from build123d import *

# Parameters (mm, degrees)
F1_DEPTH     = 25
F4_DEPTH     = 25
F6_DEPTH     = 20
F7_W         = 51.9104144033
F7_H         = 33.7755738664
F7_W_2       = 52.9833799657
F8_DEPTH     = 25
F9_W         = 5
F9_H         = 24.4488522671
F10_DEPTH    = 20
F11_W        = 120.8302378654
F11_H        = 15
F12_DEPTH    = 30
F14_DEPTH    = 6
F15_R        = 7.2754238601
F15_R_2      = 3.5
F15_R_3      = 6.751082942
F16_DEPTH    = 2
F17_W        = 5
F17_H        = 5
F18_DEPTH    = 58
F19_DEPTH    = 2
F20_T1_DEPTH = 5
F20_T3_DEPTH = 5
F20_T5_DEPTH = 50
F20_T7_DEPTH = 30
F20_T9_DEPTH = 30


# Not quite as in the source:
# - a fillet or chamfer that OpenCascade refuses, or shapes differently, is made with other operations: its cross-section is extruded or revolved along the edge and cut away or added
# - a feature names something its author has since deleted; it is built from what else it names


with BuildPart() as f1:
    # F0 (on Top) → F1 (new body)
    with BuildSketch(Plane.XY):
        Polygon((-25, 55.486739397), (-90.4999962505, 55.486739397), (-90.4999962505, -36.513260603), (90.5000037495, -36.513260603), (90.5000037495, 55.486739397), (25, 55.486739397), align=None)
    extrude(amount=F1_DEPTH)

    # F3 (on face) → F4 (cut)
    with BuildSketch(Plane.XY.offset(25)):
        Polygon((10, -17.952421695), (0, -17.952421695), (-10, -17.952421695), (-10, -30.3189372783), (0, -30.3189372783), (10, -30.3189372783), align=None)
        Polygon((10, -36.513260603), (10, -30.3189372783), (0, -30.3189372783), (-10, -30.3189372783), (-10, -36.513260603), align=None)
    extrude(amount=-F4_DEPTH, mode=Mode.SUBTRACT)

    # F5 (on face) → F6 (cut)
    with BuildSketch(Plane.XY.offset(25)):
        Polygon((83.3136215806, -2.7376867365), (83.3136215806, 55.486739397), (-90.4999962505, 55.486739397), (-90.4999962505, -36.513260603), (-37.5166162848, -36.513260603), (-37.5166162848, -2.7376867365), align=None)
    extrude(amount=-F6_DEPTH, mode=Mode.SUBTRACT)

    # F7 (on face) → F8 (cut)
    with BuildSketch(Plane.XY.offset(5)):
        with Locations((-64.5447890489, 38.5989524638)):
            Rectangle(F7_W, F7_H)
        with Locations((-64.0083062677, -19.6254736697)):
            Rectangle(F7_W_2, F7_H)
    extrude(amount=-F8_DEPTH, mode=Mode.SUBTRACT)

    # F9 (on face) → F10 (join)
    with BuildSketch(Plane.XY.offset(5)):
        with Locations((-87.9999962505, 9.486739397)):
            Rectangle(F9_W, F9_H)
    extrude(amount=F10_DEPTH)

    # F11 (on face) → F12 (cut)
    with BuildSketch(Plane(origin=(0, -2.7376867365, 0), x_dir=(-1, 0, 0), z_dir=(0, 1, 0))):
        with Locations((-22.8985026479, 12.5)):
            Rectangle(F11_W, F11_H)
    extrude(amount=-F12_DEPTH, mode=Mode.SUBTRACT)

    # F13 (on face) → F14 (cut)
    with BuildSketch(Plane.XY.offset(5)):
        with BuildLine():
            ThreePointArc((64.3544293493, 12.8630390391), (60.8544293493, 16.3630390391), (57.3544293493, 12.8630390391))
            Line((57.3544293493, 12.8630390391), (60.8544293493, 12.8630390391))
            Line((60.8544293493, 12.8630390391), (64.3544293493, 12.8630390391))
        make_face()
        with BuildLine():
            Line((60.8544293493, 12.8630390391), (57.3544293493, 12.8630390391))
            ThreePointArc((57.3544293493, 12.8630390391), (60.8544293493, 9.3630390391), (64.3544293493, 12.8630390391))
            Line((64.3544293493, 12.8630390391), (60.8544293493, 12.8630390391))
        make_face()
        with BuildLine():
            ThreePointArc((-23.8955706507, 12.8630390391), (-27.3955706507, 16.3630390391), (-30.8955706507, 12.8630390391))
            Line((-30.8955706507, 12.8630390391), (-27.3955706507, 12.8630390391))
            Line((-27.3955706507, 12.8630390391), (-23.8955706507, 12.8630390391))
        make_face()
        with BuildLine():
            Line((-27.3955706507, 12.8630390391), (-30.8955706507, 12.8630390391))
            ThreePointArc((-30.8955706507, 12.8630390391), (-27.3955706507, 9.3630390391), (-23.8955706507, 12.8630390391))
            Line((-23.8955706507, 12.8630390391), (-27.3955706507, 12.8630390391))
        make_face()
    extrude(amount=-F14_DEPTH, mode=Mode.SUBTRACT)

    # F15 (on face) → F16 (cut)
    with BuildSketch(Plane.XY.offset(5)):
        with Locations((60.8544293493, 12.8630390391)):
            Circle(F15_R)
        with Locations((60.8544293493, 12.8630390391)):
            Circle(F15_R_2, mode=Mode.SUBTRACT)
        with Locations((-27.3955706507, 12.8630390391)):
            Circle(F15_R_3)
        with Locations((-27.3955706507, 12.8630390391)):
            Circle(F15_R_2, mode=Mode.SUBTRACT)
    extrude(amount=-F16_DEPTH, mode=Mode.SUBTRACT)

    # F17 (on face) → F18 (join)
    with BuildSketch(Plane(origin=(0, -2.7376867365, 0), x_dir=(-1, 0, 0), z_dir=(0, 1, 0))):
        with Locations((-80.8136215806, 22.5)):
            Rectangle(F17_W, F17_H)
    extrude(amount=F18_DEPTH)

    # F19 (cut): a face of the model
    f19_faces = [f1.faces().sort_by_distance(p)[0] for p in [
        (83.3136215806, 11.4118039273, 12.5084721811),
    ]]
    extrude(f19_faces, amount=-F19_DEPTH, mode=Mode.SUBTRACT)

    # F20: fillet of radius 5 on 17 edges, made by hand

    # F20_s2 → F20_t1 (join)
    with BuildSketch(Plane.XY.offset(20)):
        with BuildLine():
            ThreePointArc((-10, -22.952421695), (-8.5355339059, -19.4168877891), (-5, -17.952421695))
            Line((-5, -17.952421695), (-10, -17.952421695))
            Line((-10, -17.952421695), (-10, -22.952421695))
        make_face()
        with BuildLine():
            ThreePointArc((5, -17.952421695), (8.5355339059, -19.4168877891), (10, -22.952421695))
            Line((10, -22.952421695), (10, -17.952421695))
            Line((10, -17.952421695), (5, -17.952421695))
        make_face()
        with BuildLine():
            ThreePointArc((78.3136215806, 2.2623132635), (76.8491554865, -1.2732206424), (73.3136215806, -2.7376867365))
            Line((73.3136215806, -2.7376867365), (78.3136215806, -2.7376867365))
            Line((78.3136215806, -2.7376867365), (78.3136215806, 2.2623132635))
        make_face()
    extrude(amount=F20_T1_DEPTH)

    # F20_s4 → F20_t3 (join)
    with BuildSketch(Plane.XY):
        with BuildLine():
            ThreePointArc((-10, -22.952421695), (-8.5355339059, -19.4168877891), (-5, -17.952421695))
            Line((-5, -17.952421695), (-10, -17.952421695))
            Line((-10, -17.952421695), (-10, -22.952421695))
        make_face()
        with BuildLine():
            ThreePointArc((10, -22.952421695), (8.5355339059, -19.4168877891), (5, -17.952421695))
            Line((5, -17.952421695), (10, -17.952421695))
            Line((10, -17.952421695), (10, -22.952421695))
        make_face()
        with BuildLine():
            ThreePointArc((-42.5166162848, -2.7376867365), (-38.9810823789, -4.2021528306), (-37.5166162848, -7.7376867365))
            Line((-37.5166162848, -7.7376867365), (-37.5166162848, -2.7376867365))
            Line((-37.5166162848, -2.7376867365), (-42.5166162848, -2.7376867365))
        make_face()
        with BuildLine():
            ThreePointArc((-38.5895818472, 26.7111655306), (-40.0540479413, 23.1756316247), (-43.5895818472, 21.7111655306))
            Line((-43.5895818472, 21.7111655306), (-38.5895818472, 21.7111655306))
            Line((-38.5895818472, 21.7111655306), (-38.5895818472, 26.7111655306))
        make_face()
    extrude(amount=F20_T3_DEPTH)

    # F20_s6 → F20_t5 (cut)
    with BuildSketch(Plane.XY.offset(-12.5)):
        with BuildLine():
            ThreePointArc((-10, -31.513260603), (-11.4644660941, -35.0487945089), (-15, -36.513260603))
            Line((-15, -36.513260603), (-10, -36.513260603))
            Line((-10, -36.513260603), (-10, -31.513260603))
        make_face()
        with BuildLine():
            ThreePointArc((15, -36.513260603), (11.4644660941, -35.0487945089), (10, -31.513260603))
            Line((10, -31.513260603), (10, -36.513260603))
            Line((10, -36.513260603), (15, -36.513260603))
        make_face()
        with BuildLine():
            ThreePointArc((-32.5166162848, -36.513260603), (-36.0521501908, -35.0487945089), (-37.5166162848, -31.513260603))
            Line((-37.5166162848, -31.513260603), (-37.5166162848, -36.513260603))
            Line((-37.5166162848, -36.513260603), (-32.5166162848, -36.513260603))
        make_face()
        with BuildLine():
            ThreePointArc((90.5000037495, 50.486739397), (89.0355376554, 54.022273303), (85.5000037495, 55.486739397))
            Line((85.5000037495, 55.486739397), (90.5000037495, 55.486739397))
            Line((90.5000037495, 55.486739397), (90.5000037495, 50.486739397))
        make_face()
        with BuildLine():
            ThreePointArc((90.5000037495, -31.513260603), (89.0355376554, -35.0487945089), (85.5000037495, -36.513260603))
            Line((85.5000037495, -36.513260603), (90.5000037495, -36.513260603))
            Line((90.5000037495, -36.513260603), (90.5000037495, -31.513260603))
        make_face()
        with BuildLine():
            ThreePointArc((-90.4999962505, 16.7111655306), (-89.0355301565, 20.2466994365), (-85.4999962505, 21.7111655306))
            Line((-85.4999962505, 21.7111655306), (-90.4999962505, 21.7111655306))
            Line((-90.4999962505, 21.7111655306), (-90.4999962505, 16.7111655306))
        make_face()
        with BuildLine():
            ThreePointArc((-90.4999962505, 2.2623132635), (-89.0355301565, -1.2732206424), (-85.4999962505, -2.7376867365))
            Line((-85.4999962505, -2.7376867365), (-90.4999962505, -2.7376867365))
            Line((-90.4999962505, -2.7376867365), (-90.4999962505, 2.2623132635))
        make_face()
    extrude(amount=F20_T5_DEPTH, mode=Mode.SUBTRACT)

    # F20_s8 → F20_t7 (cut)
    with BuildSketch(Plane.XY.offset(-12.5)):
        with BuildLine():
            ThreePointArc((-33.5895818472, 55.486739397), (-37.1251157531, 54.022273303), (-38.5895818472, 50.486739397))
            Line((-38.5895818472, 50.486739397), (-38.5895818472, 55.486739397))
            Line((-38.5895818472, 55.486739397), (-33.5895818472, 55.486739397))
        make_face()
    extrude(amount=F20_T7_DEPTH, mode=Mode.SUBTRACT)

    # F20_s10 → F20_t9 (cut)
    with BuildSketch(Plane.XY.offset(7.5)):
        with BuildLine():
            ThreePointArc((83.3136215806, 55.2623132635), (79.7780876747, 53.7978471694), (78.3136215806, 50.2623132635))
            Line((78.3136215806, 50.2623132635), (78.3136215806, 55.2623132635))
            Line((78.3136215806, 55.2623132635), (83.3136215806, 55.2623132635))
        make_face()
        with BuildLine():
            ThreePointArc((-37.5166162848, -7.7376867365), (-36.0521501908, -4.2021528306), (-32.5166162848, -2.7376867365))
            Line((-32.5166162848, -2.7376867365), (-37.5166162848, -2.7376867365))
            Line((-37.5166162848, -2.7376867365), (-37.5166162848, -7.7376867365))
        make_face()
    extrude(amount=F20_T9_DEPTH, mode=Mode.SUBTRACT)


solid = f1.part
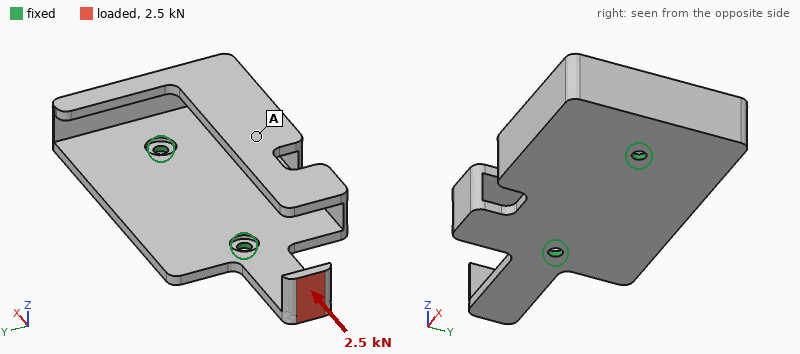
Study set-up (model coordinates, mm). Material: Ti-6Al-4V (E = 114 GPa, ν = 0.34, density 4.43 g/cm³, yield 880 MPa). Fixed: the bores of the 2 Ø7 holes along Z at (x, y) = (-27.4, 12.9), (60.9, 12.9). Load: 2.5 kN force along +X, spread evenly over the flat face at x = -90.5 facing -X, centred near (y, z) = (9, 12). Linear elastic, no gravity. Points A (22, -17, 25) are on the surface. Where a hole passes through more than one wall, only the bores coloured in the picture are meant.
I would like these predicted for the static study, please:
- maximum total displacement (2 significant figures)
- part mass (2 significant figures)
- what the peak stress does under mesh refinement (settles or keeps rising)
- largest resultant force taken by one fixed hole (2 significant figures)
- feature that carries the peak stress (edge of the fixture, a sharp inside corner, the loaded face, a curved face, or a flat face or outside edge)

2.1 mm
450 g
keeps rising
1.3 kN
edge of the fixture
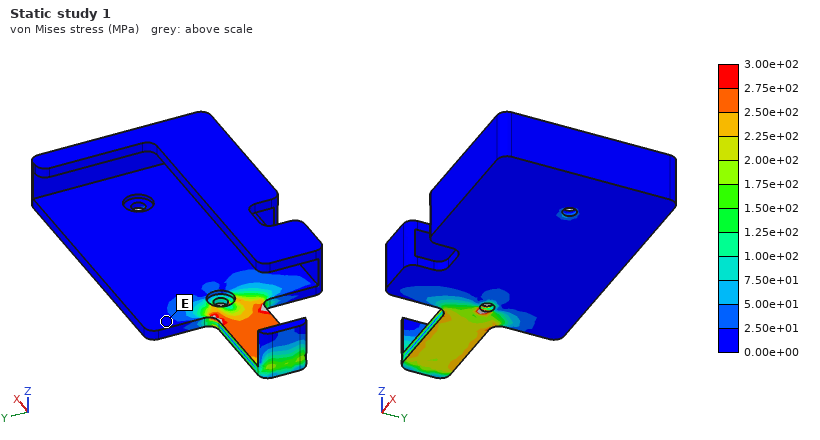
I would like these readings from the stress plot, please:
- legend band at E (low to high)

0.00e+00 to 2.50e+01 MPa
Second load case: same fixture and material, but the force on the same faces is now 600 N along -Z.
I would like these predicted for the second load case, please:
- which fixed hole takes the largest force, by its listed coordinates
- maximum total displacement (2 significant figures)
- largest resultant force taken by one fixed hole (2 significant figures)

(-27.4, 12.9)
1.9 mm
1.4 kN
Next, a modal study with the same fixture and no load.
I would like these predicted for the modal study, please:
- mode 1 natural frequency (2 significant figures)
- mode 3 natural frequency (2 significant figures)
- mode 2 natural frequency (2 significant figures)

640 Hz
1000 Hz
710 Hz
